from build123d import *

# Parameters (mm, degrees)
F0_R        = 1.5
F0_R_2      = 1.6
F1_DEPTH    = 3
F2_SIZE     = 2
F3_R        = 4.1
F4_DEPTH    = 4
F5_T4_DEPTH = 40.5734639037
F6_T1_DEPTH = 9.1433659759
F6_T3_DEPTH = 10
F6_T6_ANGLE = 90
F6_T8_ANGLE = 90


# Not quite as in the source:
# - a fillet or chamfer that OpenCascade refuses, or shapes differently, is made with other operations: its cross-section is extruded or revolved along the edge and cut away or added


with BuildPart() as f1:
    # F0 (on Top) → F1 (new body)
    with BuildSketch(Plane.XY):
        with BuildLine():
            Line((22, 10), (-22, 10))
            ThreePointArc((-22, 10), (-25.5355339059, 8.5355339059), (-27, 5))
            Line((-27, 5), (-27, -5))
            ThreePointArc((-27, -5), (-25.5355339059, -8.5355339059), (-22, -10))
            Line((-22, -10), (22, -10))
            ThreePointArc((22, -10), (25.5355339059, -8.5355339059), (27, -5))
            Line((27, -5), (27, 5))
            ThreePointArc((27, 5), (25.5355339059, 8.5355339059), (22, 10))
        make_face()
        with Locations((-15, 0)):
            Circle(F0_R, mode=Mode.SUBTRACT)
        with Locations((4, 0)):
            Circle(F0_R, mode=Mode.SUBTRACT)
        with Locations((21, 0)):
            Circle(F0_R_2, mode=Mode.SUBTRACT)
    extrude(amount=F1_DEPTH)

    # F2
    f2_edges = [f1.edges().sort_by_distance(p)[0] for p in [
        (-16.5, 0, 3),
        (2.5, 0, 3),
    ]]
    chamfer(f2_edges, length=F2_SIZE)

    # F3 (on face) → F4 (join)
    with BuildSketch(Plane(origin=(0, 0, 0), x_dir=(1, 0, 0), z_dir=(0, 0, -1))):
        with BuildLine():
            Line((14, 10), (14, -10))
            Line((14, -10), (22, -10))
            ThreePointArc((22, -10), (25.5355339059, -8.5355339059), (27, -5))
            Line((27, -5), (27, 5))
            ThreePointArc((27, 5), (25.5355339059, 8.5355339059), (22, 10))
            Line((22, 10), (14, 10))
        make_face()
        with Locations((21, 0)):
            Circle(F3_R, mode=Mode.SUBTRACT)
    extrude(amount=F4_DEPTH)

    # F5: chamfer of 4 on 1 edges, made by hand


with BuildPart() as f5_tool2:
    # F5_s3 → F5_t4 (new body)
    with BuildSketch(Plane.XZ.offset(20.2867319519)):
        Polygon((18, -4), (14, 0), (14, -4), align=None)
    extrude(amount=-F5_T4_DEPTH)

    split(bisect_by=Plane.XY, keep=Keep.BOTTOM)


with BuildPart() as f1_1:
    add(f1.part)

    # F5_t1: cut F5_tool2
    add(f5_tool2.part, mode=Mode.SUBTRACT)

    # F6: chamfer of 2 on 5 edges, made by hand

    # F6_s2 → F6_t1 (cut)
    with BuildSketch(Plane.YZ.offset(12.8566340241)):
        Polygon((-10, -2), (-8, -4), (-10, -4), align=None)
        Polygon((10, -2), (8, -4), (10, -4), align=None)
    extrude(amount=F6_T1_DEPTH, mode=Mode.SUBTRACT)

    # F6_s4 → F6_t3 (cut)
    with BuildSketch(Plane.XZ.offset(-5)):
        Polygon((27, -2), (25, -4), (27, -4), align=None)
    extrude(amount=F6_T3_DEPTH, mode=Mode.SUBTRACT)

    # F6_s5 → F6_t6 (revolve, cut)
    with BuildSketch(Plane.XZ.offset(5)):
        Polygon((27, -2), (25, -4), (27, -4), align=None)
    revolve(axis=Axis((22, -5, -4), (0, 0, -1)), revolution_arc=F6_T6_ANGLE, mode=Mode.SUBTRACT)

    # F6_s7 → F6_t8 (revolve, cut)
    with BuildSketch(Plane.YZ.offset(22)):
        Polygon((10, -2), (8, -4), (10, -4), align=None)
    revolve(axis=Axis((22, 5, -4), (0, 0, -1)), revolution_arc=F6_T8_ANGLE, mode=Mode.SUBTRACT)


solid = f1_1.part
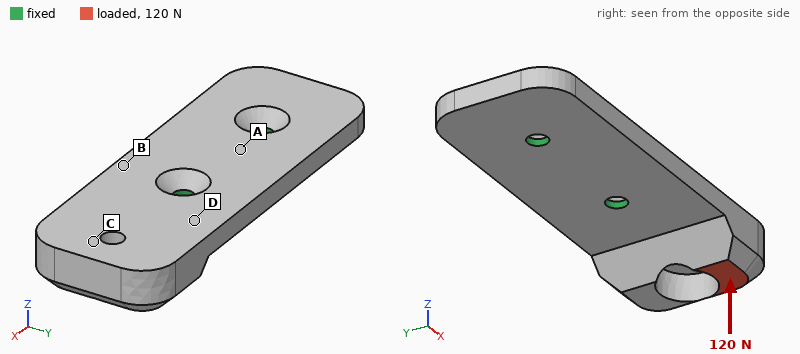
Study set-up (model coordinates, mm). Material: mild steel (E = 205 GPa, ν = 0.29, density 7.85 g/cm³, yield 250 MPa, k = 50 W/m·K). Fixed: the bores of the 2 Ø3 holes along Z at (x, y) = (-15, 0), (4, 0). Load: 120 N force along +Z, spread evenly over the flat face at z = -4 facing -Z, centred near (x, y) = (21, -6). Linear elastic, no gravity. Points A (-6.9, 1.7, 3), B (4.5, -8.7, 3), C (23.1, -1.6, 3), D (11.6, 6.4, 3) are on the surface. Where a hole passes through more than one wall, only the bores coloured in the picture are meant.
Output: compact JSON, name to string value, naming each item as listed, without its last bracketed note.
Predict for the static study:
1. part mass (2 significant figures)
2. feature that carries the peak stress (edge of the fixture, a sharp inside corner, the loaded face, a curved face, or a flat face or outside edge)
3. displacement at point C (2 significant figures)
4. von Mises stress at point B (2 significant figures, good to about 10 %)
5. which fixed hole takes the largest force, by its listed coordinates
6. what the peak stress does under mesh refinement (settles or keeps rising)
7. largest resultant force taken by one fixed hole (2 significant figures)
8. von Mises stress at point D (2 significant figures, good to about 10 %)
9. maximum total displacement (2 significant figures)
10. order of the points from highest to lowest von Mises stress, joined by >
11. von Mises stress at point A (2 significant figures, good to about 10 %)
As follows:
{"part mass": "28 g", "feature that carries the peak stress": "edge of the fixture", "displacement at point C": "43 µm", "von Mises stress at point B": "63 MPa", "which fixed hole takes the largest force, by its listed coordinates": "(4, 0)", "what the peak stress does under mesh refinement": "keeps rising", "largest resultant force taken by one fixed hole": "320 N", "von Mises stress at point D": "50 MPa", "maximum total displacement": "58 µm", "order of the points from highest to lowest von Mises stress, joined by >": "B > D > A > C", "von Mises stress at point A": "17 MPa"}
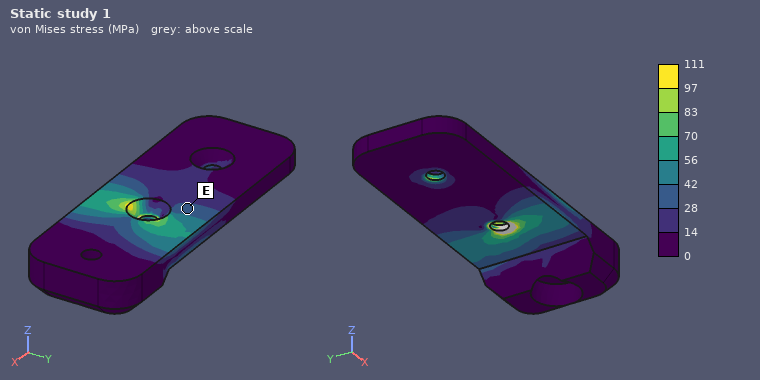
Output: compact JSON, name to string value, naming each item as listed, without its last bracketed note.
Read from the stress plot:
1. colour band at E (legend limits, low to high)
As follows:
{"colour band at E": "28 to 42 MPa"}
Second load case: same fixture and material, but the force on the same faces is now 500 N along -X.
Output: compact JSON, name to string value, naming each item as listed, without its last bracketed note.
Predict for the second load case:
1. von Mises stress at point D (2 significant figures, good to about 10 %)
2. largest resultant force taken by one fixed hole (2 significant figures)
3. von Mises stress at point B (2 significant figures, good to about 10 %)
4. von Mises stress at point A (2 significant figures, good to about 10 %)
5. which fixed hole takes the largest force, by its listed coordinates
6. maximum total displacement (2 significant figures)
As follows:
{"von Mises stress at point D": "87 MPa", "largest resultant force taken by one fixed hole": "710 N", "von Mises stress at point B": "61 MPa", "von Mises stress at point A": "22 MPa", "which fixed hole takes the largest force, by its listed coordinates": "(4, 0)", "maximum total displacement": "85 µm"}
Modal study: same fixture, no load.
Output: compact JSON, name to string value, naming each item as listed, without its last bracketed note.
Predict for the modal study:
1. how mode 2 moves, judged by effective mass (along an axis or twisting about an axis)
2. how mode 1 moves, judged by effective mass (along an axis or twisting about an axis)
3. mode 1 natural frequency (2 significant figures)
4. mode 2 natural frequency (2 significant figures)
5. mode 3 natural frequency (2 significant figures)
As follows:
{"how mode 2 moves, judged by effective mass": "twisting about X", "how mode 1 moves, judged by effective mass": "along Z", "mode 1 natural frequency": "2900 Hz", "mode 2 natural frequency": "5700 Hz", "mode 3 natural frequency": "10 kHz"}
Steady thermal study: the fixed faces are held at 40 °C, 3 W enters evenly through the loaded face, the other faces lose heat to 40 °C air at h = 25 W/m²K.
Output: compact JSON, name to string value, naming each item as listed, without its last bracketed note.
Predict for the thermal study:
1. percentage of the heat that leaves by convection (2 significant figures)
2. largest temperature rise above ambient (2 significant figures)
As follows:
{"percentage of the heat that leaves by convection": "16 %", "largest temperature rise above ambient": "25 K"}
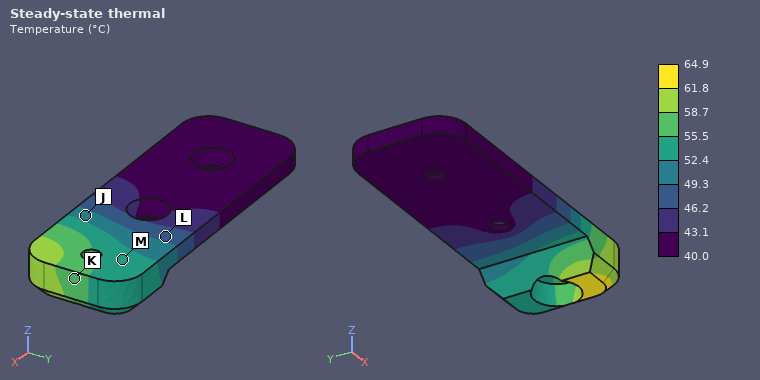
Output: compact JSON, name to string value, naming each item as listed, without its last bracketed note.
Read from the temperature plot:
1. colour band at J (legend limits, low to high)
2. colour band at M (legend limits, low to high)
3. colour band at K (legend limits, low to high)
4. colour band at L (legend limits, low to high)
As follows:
{"colour band at J": "49.3 to 52.4 °C", "colour band at M": "52.4 to 55.5 °C", "colour band at K": "55.5 to 58.7 °C", "colour band at L": "46.2 to 49.3 °C"}
